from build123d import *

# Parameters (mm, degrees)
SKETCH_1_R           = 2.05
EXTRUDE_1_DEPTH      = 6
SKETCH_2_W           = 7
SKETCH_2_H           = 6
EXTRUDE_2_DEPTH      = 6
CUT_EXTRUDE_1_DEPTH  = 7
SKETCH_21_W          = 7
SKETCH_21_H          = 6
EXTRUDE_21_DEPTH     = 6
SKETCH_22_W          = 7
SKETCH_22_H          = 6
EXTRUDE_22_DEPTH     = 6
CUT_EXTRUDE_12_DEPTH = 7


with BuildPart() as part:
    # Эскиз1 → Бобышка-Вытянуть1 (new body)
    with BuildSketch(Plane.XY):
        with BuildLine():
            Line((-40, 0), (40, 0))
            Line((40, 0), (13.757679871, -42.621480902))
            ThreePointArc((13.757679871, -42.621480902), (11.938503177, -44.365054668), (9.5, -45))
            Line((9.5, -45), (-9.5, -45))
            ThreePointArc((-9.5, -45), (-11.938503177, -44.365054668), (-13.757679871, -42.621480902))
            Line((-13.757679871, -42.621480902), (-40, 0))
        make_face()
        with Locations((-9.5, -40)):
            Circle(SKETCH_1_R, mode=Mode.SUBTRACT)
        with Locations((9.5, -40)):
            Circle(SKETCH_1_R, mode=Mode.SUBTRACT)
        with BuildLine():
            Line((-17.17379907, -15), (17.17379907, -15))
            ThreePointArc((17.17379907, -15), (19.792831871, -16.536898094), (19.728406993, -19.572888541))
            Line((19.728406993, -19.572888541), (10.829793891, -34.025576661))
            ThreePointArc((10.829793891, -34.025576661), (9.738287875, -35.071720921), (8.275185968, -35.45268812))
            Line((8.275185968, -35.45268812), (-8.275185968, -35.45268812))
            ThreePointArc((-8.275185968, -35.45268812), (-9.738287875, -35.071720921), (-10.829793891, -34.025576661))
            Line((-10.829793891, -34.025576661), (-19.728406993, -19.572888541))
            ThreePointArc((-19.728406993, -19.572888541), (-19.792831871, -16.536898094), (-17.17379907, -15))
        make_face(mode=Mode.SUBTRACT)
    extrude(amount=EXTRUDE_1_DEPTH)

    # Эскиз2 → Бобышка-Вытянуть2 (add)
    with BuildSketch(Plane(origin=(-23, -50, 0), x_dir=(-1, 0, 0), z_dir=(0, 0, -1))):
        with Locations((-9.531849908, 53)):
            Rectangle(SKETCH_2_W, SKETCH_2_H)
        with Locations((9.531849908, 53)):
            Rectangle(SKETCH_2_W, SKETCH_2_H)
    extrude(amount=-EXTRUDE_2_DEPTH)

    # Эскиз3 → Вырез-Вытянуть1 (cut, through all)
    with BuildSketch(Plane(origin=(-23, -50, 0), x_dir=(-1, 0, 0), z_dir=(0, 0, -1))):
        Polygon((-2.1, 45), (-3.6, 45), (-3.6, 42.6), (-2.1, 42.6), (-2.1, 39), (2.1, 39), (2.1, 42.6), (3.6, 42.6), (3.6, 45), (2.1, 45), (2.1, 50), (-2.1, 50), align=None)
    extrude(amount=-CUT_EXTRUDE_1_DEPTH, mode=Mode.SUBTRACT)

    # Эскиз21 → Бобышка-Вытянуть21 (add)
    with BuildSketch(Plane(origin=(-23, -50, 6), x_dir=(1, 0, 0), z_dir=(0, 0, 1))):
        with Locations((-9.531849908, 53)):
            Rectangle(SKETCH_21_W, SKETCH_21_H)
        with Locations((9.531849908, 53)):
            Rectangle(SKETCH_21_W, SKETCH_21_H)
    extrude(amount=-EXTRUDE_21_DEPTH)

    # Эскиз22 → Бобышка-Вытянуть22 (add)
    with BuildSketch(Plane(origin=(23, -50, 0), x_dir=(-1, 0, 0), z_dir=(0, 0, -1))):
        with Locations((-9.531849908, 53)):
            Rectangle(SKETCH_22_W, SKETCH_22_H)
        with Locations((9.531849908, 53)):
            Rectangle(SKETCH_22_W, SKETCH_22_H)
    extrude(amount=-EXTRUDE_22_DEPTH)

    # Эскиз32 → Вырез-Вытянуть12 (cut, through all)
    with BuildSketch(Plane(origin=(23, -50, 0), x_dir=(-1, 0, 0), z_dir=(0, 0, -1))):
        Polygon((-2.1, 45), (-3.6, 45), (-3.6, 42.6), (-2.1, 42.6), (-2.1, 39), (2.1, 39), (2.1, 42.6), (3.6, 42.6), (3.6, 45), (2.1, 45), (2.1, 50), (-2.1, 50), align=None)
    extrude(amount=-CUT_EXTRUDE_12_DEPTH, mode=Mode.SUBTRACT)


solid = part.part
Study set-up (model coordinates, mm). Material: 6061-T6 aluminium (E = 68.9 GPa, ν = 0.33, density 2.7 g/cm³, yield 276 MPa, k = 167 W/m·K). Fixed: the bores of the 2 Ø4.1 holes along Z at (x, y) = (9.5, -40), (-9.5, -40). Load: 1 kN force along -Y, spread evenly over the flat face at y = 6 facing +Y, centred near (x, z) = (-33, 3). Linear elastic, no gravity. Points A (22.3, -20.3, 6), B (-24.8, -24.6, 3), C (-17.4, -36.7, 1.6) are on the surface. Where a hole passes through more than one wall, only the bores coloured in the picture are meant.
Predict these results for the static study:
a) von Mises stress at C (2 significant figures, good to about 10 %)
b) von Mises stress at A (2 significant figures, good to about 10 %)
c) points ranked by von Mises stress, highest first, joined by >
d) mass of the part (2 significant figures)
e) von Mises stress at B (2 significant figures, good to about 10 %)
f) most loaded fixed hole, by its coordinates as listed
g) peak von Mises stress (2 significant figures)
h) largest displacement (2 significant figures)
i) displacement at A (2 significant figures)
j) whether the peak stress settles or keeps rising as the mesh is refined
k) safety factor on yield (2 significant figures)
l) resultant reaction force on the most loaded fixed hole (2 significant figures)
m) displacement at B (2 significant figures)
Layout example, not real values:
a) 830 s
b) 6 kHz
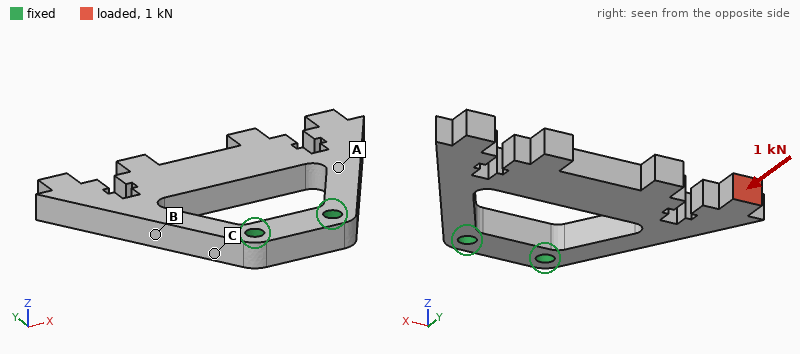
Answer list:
a) 150 MPa
b) 29 MPa
c) C > B > A
d) 28 g
e) 57 MPa
f) (-9.5, -40)
g) 220 MPa
h) 0.44 mm
i) 0.13 mm
j) settles
k) 1.2
l) 1.5 kN
m) 0.12 mm
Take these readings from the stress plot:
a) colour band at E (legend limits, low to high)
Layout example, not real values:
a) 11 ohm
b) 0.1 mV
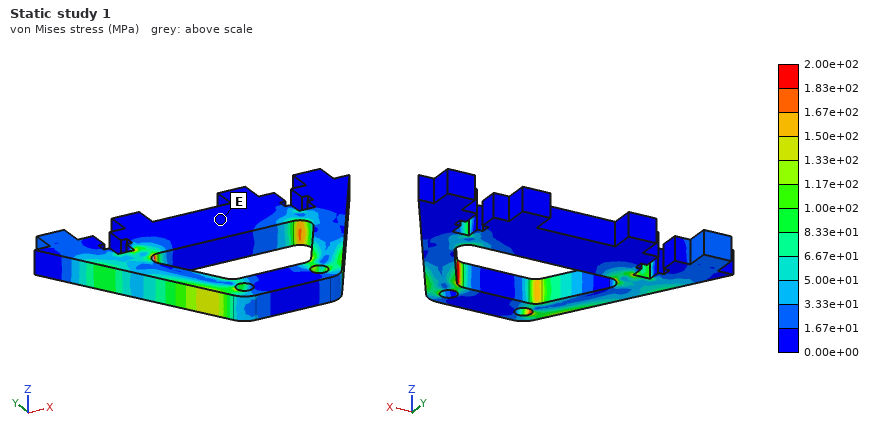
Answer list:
a) 0.00e+00 to 1.67e+01 MPa
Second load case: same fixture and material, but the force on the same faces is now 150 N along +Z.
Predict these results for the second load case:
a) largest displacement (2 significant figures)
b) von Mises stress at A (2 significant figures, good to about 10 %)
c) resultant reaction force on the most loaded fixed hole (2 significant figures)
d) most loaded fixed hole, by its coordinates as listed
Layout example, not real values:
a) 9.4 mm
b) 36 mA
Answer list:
a) 0.58 mm
b) 45 MPa
c) 170 N
d) (-9.5, -40)
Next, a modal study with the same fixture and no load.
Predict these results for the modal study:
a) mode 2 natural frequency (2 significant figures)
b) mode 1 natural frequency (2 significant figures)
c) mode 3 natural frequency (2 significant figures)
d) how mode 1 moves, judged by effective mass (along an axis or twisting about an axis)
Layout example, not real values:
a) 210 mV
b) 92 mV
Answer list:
a) 1900 Hz
b) 1200 Hz
c) 1900 Hz
d) along Z
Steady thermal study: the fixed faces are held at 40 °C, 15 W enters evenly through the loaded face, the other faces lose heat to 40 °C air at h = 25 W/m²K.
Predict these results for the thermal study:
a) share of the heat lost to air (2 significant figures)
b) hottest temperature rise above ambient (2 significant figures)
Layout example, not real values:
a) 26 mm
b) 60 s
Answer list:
a) 20 %
b) 75 K
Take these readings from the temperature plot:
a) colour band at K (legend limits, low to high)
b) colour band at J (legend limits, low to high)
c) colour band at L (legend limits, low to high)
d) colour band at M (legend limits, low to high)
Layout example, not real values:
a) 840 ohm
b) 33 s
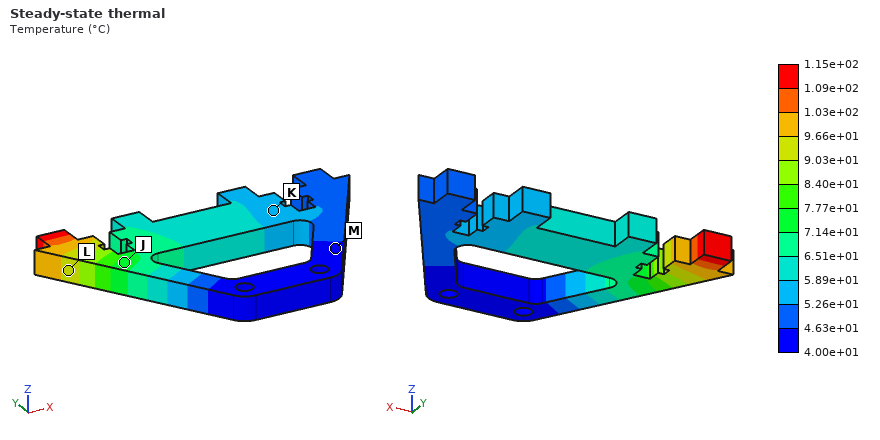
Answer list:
a) 5.26e+01 to 5.89e+01 °C
b) 7.14e+01 to 7.77e+01 °C
c) 9.03e+01 to 9.66e+01 °C
d) 4.00e+01 to 4.63e+01 °C
